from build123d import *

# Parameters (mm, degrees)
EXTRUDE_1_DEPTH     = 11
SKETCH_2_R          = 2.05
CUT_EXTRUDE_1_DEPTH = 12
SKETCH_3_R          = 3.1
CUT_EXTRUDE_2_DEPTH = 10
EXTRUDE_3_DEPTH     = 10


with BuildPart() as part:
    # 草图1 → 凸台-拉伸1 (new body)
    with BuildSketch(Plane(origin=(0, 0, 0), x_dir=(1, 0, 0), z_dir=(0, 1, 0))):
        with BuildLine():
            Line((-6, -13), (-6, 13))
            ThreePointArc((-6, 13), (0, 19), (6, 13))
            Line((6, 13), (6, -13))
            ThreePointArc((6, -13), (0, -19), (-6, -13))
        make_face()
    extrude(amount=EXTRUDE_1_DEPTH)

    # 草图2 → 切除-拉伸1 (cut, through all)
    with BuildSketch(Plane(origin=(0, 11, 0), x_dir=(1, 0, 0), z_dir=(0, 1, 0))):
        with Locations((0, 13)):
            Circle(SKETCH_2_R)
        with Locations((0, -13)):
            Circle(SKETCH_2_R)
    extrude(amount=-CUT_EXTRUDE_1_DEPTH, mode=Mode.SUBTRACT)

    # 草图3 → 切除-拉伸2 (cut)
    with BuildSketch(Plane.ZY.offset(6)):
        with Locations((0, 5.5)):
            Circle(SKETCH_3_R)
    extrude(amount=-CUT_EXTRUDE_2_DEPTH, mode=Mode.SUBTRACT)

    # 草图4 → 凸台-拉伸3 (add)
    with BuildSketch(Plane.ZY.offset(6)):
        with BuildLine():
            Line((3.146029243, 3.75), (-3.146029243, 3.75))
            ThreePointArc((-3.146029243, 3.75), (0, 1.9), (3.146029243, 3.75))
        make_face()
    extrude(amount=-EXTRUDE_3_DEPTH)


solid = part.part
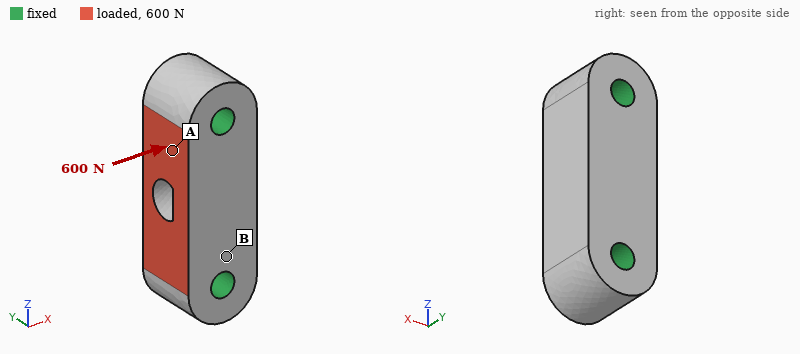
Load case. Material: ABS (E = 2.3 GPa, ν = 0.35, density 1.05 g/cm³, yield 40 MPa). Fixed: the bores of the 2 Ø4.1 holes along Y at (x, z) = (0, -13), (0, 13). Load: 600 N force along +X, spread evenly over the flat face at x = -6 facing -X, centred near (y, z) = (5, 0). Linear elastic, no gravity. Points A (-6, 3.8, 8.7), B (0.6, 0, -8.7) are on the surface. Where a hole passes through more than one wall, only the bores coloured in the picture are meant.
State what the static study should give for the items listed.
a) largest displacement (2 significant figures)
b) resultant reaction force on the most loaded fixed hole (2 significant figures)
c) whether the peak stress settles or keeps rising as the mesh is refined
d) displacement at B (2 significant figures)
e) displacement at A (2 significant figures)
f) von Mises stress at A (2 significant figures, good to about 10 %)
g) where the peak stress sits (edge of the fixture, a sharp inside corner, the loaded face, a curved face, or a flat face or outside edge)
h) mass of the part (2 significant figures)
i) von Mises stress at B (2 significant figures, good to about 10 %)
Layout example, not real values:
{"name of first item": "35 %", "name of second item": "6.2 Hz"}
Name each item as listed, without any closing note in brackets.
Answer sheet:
{"largest displacement": "37 µm", "resultant reaction force on the most loaded fixed hole": "300 N", "whether the peak stress settles or keeps rising as the mesh is refined": "keeps rising", "displacement at B": "13 µm", "displacement at A": "21 µm", "von Mises stress at A": "2.1 MPa", "where the peak stress sits": "edge of the fixture", "mass of the part": "4.3 g", "von Mises stress at B": "4.2 MPa"}
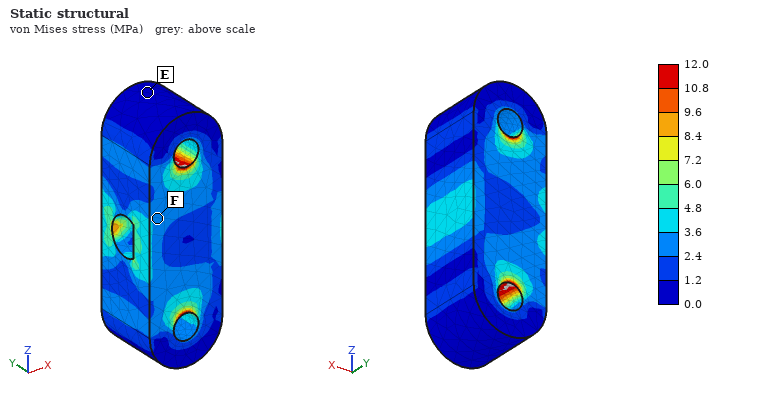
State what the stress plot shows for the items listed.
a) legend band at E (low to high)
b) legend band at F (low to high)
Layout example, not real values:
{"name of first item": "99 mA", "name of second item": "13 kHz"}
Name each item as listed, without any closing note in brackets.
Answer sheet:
{"legend band at E": "0.0 to 1.2 MPa", "legend band at F": "2.4 to 3.6 MPa"}
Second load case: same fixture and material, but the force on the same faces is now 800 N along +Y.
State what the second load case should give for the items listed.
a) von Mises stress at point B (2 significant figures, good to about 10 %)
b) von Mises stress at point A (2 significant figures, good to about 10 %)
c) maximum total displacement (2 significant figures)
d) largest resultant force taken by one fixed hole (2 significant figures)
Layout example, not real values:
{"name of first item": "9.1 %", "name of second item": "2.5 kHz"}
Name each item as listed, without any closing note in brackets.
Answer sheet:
{"von Mises stress at point B": "7.7 MPa", "von Mises stress at point A": "12 MPa", "maximum total displacement": "0.11 mm", "largest resultant force taken by one fixed hole": "400 N"}
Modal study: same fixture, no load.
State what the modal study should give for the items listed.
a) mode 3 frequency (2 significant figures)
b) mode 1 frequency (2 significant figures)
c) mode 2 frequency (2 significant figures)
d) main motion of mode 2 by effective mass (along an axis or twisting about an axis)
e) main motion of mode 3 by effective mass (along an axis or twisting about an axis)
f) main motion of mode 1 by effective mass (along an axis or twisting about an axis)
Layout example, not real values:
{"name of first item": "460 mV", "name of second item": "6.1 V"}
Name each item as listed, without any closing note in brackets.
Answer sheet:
{"mode 3 frequency": "17 kHz", "mode 1 frequency": "13 kHz", "mode 2 frequency": "15 kHz", "main motion of mode 2 by effective mass": "along Y", "main motion of mode 3 by effective mass": "twisting about Z", "main motion of mode 1 by effective mass": "along X"}
